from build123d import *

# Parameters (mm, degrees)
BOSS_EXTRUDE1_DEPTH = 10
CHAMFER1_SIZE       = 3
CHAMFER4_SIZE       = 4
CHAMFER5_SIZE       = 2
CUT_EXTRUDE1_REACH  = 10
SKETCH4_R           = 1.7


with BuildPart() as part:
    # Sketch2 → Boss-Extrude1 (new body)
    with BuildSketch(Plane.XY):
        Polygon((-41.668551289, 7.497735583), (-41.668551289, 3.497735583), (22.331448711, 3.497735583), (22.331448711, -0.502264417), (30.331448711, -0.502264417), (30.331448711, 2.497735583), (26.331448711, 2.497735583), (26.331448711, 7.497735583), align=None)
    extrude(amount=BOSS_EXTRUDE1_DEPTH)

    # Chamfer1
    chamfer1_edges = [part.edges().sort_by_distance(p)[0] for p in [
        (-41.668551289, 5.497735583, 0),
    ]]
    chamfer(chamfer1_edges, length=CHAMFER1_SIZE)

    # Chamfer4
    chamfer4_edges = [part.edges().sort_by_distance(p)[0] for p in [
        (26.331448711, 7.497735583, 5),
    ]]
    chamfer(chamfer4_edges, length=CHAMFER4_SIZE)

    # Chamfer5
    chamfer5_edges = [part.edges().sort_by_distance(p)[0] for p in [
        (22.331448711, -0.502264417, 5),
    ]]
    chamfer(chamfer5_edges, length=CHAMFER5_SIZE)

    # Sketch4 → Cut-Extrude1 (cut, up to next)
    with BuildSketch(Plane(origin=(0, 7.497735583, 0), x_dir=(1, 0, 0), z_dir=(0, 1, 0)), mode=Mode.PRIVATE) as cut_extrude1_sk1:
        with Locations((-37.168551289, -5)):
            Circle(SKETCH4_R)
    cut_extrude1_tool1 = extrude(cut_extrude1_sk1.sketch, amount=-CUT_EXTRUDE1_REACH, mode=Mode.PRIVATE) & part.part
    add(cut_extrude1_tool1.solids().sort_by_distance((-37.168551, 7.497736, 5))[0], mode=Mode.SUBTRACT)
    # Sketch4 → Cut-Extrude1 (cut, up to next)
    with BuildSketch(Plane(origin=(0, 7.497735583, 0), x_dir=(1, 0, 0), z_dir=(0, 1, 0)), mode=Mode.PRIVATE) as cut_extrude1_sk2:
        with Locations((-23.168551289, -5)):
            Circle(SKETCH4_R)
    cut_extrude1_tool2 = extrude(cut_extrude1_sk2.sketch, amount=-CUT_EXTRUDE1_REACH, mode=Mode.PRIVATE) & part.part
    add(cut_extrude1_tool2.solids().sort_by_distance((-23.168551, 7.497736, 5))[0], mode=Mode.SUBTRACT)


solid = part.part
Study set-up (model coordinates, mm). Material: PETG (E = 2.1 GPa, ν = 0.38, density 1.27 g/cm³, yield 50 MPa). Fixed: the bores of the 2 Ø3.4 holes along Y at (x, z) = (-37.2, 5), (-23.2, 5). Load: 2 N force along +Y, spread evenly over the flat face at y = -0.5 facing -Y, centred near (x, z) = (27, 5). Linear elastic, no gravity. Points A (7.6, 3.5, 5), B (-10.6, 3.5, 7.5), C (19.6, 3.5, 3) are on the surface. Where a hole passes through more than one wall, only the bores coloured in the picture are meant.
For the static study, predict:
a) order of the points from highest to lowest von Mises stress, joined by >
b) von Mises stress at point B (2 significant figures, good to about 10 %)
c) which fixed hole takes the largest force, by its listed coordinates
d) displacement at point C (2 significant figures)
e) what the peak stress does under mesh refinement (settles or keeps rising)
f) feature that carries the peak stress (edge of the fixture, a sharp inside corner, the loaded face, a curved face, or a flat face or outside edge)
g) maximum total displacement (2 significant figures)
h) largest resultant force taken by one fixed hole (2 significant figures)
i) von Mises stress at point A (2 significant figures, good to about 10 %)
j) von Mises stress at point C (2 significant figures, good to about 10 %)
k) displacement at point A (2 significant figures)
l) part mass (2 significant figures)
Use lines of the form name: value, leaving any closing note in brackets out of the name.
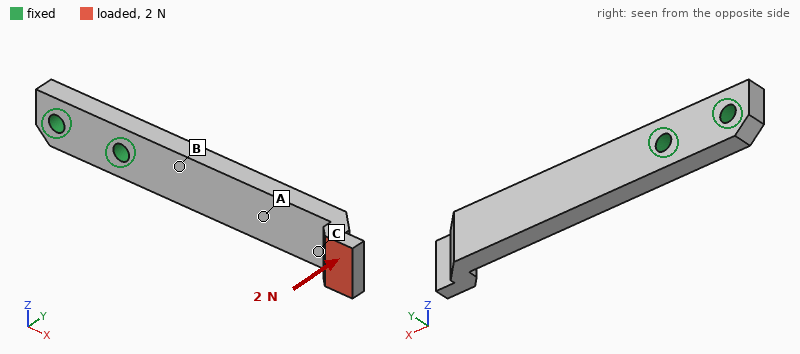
order of the points from highest to lowest von Mises stress, joined by >: B > A > C
von Mises stress at point B: 2.8 MPa
which fixed hole takes the largest force, by its listed coordinates: (-23.2, 5)
displacement at point C: 0.57 mm
what the peak stress does under mesh refinement: keeps rising
feature that carries the peak stress: edge of the fixture
maximum total displacement: 0.81 mm
largest resultant force taken by one fixed hole: 2.7 N
von Mises stress at point A: 1.5 MPa
von Mises stress at point C: 0.59 MPa
displacement at point A: 0.32 mm
part mass: 3.6 g
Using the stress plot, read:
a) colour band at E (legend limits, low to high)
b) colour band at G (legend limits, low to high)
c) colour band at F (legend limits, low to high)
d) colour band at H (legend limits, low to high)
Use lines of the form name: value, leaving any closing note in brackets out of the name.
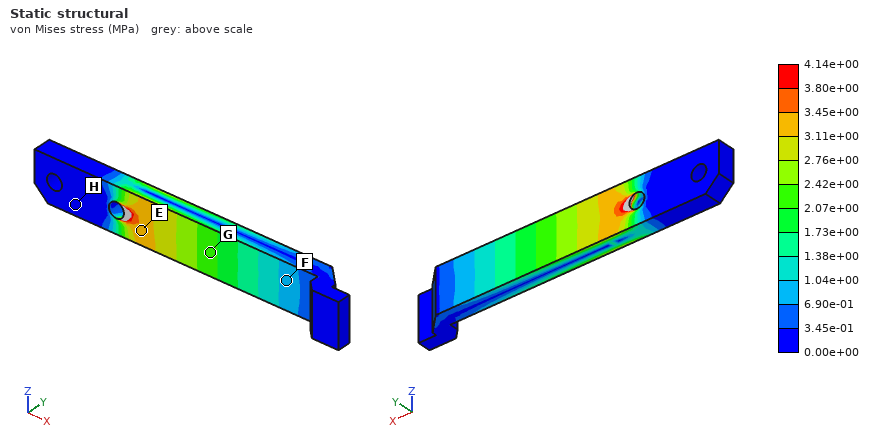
colour band at E: 3.11e+00 to 3.45e+00 MPa
colour band at G: 2.07e+00 to 2.42e+00 MPa
colour band at F: 6.90e-01 to 1.04e+00 MPa
colour band at H: 0.00e+00 to 3.45e-01 MPa
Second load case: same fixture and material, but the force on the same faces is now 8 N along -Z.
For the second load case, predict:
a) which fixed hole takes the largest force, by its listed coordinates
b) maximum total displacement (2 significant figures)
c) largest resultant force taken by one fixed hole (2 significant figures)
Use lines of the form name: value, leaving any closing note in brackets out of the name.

which fixed hole takes the largest force, by its listed coordinates: (-23.2, 5)
maximum total displacement: 0.75 mm
largest resultant force taken by one fixed hole: 21 N
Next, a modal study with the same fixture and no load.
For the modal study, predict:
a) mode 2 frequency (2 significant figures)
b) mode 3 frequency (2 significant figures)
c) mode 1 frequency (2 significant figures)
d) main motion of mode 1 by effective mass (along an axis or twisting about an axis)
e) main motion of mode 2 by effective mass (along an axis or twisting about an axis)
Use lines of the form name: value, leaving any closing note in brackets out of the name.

mode 2 frequency: 640 Hz
mode 3 frequency: 1800 Hz
mode 1 frequency: 300 Hz
main motion of mode 1 by effective mass: along Y
main motion of mode 2 by effective mass: along Z
